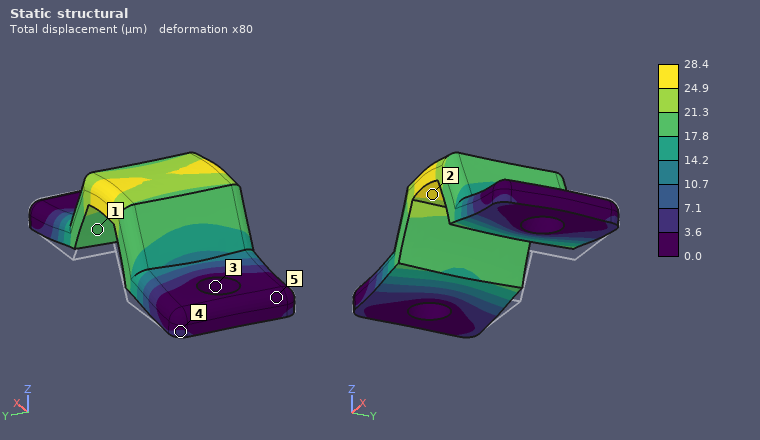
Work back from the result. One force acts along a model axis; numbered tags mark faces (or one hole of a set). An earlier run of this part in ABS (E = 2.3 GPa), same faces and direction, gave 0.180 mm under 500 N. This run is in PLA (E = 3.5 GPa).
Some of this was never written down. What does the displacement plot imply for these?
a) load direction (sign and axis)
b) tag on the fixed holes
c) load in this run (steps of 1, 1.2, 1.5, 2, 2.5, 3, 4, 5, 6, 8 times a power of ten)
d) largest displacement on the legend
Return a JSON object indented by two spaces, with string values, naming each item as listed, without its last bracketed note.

{
  "load direction": "+Z",
  "tag on the fixed holes": "3",
  "load in this run": "120 N",
  "largest displacement on the legend": "28.4 µm"
}
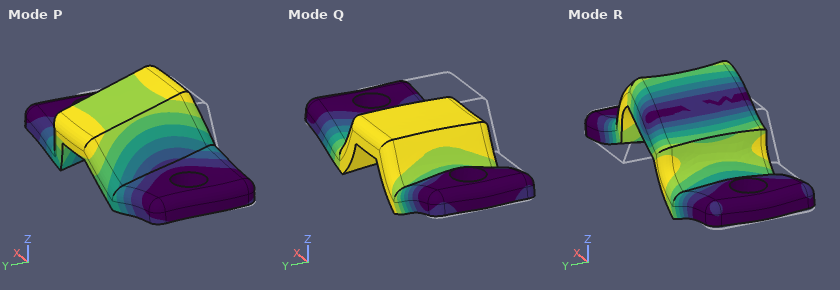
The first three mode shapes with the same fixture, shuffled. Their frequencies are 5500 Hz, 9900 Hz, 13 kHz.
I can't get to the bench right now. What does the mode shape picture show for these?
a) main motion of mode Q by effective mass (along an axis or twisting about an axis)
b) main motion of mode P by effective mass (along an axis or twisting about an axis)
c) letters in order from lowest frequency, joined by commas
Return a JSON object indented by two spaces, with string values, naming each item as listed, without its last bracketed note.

{
  "main motion of mode Q by effective mass": "along Z",
  "main motion of mode P by effective mass": "along Y",
  "letters in order from lowest frequency, joined by commas": "P, Q, R"
}
